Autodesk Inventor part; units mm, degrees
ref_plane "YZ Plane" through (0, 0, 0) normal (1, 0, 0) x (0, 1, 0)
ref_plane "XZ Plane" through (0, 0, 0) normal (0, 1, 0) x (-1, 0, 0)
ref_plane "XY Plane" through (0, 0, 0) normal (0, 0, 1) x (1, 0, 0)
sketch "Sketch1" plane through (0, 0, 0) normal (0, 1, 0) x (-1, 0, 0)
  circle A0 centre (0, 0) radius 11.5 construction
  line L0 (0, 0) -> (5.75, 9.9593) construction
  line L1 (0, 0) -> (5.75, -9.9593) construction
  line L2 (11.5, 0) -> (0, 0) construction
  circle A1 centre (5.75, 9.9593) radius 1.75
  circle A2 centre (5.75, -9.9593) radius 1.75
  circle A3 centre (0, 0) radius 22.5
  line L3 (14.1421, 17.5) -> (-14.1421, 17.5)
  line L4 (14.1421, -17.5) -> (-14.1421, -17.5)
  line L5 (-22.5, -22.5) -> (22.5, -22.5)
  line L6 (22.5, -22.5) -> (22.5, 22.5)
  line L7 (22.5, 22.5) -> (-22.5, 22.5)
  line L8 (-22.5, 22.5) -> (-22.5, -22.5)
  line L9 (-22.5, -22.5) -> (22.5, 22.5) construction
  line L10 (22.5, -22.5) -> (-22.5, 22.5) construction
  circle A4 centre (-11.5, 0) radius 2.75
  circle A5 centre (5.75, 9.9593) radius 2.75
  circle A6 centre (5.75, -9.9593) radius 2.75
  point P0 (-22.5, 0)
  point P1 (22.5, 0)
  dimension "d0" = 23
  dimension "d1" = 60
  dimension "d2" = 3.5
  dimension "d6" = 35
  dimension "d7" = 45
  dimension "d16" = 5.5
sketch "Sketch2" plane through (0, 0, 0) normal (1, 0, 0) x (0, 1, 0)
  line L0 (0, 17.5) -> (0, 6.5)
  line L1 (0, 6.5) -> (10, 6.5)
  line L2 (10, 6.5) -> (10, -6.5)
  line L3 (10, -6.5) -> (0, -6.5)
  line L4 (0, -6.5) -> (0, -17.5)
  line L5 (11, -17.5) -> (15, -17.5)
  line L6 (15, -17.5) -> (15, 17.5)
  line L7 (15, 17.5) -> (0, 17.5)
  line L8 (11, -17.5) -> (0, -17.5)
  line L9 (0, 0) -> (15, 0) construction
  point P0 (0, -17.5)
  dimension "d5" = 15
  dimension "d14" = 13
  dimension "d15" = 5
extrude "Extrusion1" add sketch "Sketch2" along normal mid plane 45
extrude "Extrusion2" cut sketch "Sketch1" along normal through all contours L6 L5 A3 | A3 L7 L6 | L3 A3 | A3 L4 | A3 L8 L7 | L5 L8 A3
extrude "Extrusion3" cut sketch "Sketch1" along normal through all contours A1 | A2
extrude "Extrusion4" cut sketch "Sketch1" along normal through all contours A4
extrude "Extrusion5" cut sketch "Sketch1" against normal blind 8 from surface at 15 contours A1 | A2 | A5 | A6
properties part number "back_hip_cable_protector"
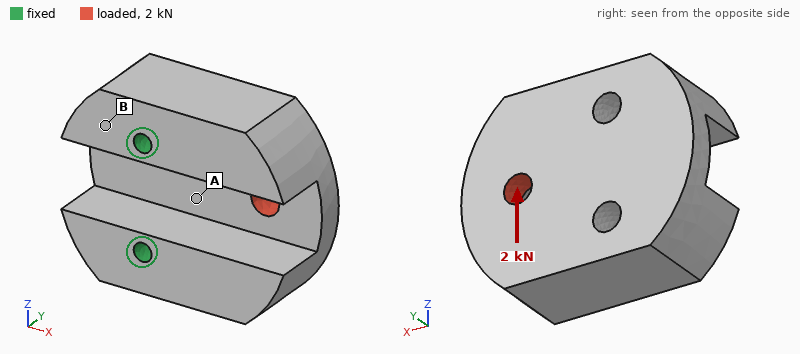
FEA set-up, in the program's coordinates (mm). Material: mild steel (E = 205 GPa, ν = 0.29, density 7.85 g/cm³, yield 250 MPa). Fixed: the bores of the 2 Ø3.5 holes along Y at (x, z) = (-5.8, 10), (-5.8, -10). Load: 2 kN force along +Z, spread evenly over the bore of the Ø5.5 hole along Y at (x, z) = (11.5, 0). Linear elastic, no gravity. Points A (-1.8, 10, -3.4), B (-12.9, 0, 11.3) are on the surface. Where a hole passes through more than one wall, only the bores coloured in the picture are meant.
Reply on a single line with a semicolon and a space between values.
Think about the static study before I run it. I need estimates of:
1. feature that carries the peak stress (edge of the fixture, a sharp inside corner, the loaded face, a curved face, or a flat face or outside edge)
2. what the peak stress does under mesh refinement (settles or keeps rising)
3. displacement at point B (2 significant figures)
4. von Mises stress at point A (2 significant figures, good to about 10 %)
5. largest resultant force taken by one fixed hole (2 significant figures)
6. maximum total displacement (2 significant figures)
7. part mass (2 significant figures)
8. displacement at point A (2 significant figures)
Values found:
edge of the fixture; keeps rising; 1.9 µm; 25 MPa; 1.7 kN; 9.4 µm; 110 g; 3.0 µm
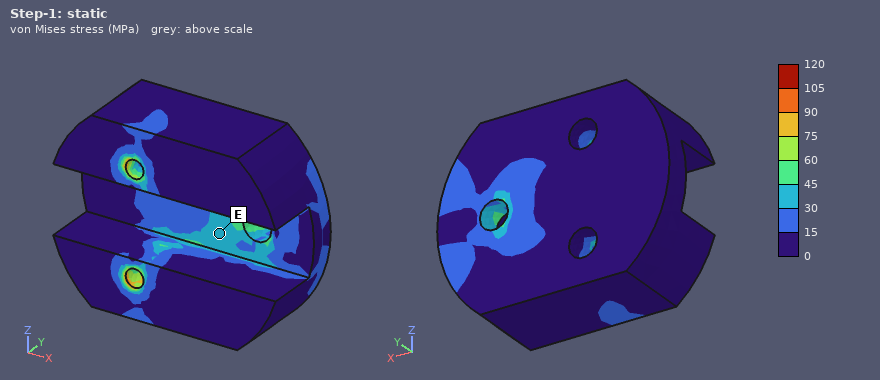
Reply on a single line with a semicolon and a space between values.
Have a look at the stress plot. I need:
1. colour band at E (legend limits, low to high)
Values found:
30 to 45 MPa
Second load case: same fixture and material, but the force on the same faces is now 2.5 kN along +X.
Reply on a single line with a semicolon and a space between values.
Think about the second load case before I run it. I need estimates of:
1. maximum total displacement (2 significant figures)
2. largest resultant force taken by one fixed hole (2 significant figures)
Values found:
15 µm; 1.3 kN
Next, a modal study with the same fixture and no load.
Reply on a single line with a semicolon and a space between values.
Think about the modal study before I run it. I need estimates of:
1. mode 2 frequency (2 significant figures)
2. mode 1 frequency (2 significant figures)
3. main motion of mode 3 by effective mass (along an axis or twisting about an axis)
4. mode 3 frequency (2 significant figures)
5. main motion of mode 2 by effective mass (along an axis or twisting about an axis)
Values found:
10 kHz; 7500 Hz; along Z; 16 kHz; along Z
